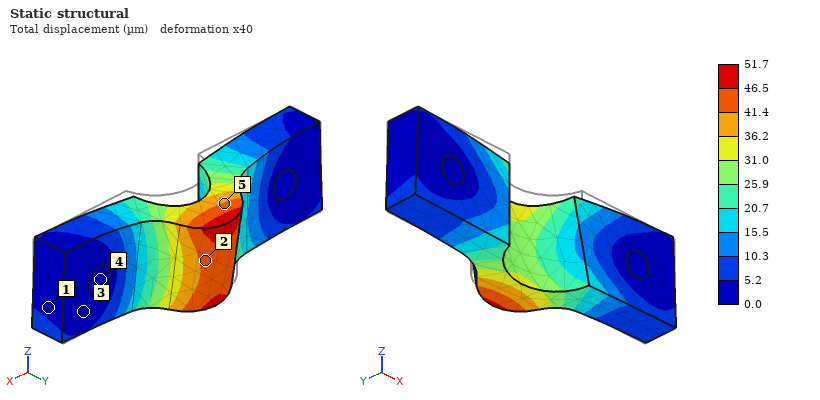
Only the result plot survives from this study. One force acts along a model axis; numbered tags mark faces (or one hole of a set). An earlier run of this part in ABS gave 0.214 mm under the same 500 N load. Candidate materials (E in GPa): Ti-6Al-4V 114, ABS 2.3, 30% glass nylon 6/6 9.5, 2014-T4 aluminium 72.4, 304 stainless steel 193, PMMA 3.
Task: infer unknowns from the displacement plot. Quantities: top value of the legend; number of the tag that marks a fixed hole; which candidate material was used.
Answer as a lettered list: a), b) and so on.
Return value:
a) 51.7 µm
b) 4
c) 30% glass nylon 6/6
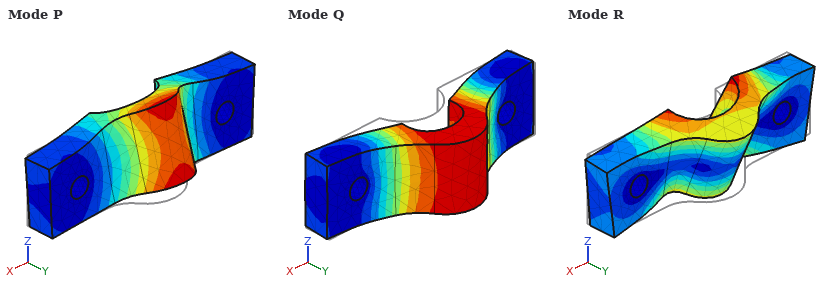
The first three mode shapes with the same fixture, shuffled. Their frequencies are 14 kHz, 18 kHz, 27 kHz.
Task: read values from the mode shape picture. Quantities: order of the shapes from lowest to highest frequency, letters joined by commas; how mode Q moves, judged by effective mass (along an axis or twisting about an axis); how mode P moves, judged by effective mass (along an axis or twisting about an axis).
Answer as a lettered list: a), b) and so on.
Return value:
a) P, Q, R
b) along Y
c) along Z
